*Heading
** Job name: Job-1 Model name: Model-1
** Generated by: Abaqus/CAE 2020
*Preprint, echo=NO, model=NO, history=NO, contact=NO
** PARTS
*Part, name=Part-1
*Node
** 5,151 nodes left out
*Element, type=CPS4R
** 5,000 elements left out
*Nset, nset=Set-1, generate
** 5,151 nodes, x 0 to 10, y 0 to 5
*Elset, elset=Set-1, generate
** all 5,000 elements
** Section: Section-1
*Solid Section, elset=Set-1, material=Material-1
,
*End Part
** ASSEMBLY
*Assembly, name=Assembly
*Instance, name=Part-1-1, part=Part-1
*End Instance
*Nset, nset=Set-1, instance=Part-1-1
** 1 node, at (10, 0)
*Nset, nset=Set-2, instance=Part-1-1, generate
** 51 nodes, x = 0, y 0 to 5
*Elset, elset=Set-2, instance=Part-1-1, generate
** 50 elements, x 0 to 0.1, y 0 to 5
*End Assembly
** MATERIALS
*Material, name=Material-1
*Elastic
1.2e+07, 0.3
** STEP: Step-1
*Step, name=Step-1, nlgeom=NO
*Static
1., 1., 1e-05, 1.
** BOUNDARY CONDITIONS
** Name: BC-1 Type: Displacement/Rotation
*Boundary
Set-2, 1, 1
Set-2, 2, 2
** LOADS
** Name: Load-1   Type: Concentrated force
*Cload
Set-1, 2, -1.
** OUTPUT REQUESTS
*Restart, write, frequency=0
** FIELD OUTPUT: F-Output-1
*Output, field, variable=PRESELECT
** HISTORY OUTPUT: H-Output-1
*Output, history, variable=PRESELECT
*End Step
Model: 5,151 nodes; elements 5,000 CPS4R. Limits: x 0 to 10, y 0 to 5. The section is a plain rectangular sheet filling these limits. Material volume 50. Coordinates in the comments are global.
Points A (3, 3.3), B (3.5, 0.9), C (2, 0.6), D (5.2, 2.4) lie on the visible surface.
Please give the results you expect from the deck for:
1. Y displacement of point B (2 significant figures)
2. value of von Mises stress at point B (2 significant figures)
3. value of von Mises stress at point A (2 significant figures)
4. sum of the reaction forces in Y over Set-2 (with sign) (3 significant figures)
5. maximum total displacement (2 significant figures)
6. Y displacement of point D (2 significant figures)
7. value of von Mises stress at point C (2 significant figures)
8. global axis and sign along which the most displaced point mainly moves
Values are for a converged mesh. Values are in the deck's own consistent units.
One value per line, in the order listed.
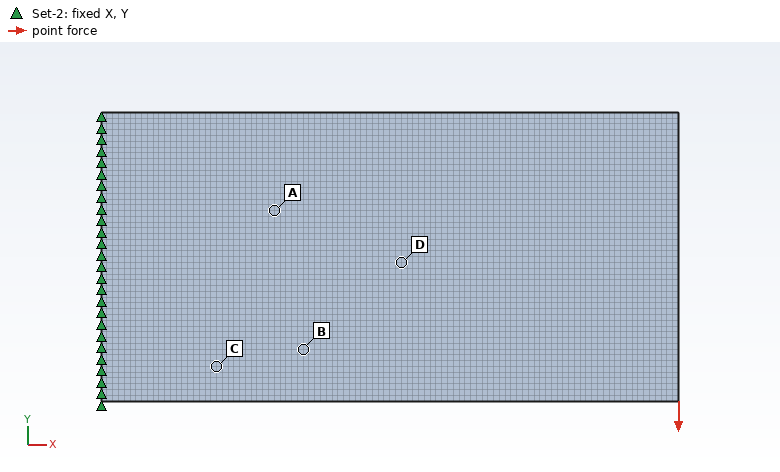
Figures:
-6.1e-07
1.0
0.72
1.00
4.3e-06
-1.1e-06
1.5
-Y
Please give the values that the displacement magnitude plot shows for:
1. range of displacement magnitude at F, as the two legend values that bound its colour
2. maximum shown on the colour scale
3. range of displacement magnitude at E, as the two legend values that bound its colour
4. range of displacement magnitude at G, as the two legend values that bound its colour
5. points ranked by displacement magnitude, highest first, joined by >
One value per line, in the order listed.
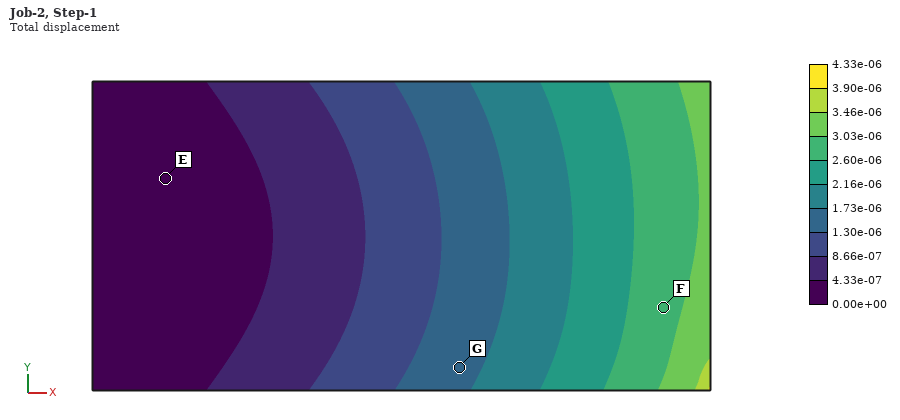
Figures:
2.60e-06 to 3.03e-06
4.33e-06
0.00e+00 to 4.33e-07
1.30e-06 to 1.73e-06
F > G > E
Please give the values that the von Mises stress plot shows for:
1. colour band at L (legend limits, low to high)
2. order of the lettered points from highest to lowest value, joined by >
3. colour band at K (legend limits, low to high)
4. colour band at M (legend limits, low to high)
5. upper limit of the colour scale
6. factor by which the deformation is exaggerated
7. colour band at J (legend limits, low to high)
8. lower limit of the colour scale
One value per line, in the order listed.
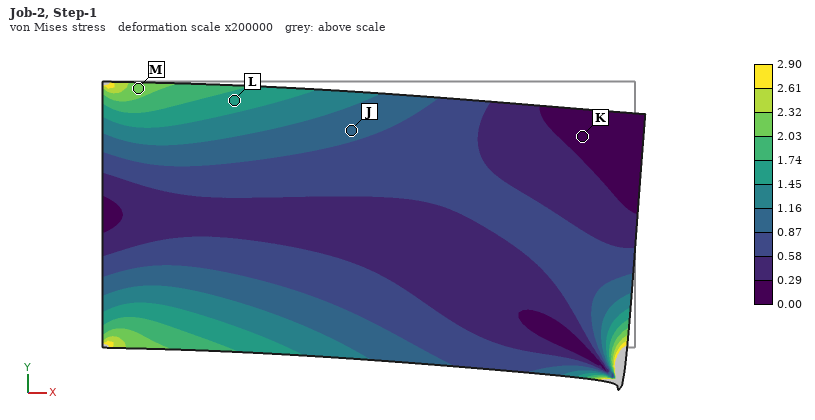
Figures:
1.45 to 1.74
M > L > J > K
0.00 to 0.29
2.03 to 2.32
2.90
200000
0.87 to 1.16
0.00
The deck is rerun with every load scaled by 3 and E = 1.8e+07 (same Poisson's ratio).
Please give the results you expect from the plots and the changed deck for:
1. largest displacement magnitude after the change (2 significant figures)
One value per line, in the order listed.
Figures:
8.7e-06
